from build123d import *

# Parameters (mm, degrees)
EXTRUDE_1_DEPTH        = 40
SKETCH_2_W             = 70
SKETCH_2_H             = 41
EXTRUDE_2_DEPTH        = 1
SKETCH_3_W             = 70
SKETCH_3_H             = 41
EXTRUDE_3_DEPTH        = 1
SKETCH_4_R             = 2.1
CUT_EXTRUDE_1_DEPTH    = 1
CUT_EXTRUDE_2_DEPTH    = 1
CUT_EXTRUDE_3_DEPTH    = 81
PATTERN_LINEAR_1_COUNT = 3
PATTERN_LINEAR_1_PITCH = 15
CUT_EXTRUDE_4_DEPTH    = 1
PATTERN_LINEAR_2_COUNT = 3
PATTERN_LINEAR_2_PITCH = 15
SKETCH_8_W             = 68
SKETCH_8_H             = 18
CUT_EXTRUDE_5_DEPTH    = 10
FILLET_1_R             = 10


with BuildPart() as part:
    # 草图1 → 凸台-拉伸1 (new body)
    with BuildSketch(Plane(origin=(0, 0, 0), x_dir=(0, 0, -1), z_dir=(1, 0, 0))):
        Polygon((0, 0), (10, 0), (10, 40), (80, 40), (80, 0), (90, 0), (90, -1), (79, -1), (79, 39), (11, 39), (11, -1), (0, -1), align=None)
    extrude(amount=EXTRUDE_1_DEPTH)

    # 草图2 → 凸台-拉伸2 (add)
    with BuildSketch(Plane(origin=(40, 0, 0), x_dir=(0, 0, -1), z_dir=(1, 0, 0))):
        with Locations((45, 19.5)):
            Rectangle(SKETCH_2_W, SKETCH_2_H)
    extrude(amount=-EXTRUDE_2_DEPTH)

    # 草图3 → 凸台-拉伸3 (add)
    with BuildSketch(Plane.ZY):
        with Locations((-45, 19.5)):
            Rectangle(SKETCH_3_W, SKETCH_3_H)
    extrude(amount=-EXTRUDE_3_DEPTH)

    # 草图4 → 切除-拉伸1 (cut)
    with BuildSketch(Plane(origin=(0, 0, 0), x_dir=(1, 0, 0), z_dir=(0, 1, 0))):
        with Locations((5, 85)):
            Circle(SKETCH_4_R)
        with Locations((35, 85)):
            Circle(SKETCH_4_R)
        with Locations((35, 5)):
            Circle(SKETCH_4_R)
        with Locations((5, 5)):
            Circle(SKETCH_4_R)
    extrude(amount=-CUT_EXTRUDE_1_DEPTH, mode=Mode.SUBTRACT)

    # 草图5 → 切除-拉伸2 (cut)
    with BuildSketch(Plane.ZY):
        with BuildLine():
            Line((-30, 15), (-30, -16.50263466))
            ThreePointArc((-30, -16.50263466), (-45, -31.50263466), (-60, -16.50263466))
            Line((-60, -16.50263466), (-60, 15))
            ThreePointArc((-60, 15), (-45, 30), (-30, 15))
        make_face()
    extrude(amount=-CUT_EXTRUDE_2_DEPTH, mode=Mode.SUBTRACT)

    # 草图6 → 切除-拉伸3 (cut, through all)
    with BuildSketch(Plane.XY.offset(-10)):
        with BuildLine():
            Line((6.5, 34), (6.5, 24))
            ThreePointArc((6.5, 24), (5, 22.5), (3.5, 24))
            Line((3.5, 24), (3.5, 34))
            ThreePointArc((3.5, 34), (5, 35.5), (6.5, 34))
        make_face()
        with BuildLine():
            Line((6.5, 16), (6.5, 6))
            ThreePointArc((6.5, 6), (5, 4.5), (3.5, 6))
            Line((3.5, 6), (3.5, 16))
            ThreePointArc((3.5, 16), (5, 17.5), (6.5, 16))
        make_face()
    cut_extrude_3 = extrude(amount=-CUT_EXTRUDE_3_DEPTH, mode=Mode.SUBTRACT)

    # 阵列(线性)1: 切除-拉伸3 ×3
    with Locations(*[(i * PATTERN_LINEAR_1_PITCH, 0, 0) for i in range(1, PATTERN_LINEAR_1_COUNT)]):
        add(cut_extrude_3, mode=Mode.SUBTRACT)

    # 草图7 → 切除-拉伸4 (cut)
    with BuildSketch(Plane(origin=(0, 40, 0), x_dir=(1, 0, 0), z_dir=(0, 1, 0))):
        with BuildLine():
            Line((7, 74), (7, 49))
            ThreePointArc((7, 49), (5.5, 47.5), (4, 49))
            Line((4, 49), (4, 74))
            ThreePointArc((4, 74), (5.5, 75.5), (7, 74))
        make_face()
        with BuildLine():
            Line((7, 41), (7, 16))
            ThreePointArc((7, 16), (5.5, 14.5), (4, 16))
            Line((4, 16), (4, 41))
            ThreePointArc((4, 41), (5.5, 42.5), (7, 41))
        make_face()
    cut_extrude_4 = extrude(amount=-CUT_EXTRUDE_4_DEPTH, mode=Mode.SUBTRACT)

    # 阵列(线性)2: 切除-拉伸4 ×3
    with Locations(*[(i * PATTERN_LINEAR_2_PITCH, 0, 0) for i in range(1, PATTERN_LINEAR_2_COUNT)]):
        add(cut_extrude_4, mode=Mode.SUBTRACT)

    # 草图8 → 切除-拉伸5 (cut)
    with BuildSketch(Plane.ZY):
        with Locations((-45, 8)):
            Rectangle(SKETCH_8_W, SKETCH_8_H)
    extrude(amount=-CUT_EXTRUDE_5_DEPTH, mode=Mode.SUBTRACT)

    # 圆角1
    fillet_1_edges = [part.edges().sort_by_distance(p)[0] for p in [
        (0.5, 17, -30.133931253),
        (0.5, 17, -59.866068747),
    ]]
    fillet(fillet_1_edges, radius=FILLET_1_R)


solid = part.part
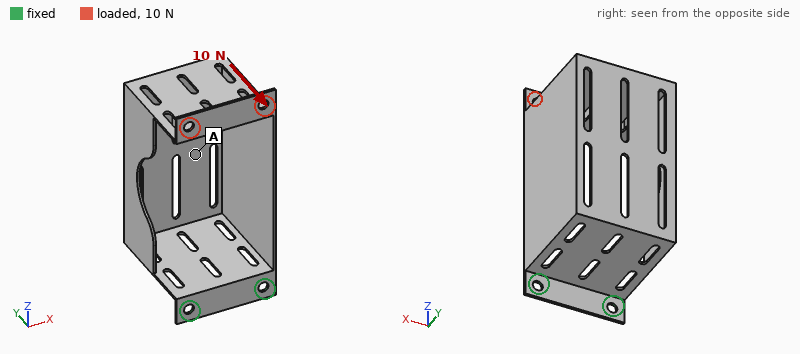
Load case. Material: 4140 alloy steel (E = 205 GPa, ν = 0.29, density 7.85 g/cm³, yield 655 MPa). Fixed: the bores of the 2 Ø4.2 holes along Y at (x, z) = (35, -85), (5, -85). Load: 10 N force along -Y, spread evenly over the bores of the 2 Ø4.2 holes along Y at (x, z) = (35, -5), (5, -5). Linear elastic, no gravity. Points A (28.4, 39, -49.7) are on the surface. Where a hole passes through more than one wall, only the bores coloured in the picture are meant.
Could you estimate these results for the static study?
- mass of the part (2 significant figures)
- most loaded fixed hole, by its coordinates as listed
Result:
76 g
(35, -85)
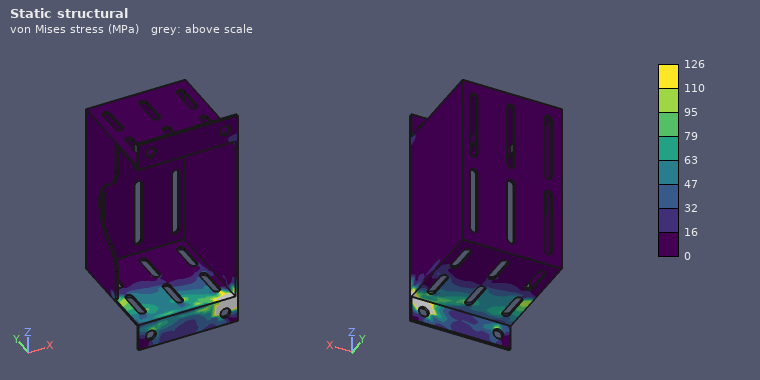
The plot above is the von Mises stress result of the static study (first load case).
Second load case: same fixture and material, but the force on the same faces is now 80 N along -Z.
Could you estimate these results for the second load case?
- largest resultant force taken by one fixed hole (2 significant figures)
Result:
42 N
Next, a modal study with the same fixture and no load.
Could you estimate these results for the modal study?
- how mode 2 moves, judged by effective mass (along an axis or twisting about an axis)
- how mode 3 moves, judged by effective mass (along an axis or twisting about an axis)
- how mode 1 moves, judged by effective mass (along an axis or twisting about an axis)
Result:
along X
along Z
along Y
